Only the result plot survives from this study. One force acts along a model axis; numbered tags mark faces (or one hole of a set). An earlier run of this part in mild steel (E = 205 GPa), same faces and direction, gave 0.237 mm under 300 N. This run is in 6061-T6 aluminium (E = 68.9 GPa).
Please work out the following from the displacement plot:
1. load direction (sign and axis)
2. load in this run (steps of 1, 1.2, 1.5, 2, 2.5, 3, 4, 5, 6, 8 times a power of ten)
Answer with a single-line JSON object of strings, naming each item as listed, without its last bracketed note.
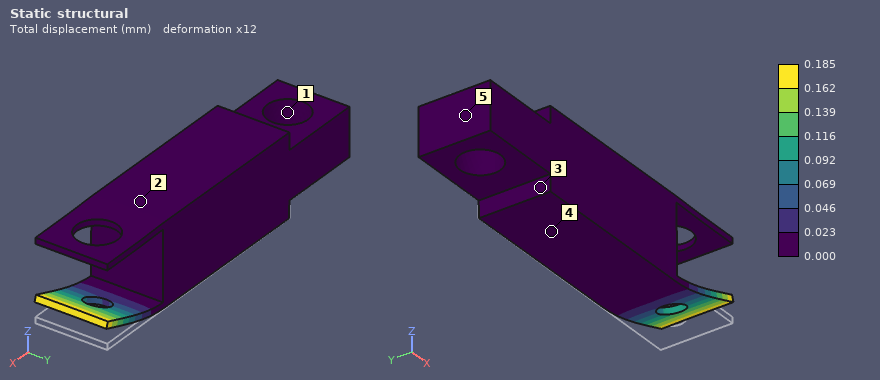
{"load direction": "+Z", "load in this run": "80 N"}
